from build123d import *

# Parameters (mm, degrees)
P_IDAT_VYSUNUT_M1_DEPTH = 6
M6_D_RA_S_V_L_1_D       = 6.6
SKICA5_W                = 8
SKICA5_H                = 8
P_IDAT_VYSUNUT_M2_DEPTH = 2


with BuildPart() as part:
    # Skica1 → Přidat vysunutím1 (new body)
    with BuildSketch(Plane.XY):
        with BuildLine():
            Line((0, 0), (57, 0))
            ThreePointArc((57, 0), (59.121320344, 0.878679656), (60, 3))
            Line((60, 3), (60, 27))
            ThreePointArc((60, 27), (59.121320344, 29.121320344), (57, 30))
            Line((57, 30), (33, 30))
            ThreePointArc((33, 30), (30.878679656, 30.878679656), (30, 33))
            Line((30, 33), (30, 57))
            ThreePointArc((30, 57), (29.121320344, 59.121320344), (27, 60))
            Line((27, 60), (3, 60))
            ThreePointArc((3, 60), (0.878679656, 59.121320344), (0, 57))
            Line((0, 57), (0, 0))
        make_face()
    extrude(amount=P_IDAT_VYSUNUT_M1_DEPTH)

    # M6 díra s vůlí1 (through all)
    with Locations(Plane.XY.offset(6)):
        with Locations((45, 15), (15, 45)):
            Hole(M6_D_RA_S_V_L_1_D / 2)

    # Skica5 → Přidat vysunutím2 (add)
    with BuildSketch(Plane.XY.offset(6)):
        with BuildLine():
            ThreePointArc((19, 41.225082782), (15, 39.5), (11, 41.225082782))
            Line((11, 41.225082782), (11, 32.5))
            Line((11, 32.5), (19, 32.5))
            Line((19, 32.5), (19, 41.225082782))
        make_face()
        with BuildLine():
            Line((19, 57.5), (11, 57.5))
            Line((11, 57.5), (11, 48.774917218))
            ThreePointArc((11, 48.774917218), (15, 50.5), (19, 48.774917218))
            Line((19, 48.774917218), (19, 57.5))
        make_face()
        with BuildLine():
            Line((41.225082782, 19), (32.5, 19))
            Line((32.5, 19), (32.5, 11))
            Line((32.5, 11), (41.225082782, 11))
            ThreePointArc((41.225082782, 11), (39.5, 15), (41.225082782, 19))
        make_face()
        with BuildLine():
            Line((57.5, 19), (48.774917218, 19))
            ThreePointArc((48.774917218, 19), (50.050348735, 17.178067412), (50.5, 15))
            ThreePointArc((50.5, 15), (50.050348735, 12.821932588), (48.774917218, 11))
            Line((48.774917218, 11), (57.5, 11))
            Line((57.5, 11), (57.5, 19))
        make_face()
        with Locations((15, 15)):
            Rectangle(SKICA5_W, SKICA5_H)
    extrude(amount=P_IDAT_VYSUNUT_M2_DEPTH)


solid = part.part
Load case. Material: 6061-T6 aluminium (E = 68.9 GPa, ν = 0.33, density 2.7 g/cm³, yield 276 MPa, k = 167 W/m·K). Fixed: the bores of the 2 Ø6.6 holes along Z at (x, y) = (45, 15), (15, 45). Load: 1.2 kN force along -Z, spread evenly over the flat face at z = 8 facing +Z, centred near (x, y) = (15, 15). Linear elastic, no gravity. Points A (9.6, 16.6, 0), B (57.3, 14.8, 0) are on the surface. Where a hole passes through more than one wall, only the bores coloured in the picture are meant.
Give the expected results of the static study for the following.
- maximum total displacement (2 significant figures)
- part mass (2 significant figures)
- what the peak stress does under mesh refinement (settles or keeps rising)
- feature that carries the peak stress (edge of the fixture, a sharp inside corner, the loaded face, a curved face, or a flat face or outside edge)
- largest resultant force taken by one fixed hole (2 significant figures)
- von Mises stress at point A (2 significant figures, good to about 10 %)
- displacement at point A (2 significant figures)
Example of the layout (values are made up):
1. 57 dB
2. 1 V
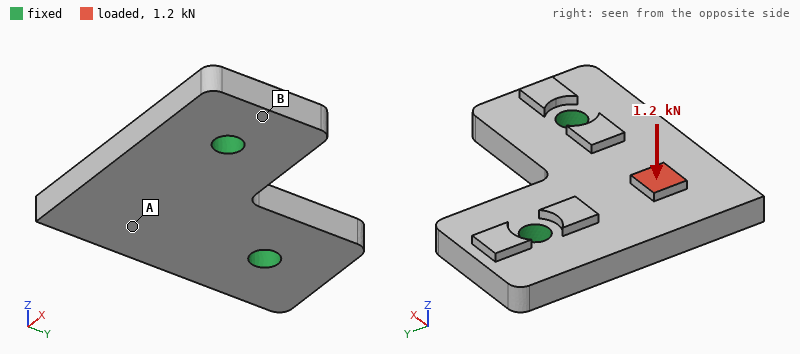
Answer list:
1. 0.18 mm
2. 44 g
3. keeps rising
4. edge of the fixture
5. 600 N
6. 31 MPa
7. 0.089 mm
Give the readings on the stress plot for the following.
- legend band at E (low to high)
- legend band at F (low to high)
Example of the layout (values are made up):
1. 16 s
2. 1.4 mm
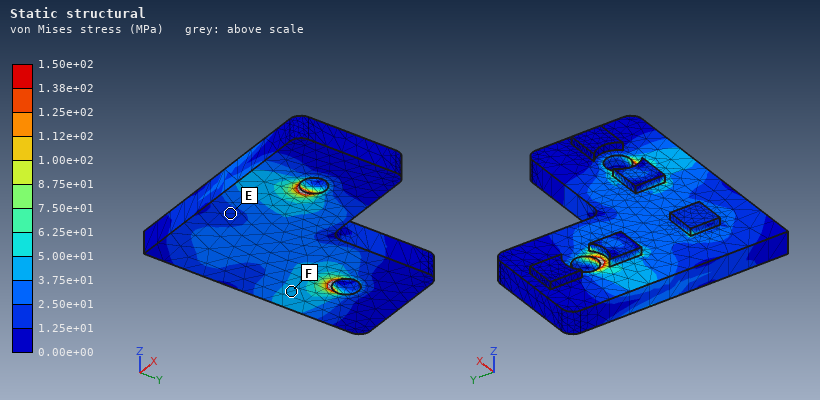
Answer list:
1. 1.25e+01 to 2.50e+01 MPa
2. 3.75e+01 to 5.00e+01 MPa
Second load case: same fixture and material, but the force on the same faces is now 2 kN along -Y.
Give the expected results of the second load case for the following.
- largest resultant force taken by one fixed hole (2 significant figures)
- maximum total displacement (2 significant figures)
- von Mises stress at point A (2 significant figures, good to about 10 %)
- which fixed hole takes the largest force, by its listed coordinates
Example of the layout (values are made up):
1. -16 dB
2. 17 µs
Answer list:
1. 1.8 kN
2. 79 µm
3. 12 MPa
4. (15, 45)
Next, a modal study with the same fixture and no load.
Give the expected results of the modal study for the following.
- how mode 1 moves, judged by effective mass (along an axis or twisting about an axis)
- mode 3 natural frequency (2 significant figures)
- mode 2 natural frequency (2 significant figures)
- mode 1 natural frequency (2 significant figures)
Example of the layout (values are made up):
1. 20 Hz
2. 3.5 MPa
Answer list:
1. along Z
2. 16 kHz
3. 14 kHz
4. 4500 Hz
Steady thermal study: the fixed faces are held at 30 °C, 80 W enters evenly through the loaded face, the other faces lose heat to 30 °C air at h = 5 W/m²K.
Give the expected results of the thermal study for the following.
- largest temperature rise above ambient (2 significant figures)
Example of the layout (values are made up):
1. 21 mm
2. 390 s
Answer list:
1. 75 K
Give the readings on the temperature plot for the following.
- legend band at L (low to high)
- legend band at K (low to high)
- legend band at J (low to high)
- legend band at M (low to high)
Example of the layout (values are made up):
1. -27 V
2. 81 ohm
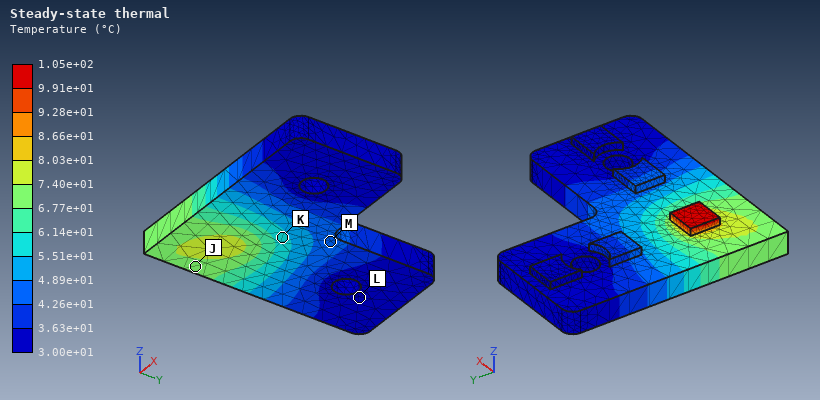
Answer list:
1. 3.00e+01 to 3.63e+01 °C
2. 5.51e+01 to 6.14e+01 °C
3. 6.77e+01 to 7.40e+01 °C
4. 4.26e+01 to 4.89e+01 °C
